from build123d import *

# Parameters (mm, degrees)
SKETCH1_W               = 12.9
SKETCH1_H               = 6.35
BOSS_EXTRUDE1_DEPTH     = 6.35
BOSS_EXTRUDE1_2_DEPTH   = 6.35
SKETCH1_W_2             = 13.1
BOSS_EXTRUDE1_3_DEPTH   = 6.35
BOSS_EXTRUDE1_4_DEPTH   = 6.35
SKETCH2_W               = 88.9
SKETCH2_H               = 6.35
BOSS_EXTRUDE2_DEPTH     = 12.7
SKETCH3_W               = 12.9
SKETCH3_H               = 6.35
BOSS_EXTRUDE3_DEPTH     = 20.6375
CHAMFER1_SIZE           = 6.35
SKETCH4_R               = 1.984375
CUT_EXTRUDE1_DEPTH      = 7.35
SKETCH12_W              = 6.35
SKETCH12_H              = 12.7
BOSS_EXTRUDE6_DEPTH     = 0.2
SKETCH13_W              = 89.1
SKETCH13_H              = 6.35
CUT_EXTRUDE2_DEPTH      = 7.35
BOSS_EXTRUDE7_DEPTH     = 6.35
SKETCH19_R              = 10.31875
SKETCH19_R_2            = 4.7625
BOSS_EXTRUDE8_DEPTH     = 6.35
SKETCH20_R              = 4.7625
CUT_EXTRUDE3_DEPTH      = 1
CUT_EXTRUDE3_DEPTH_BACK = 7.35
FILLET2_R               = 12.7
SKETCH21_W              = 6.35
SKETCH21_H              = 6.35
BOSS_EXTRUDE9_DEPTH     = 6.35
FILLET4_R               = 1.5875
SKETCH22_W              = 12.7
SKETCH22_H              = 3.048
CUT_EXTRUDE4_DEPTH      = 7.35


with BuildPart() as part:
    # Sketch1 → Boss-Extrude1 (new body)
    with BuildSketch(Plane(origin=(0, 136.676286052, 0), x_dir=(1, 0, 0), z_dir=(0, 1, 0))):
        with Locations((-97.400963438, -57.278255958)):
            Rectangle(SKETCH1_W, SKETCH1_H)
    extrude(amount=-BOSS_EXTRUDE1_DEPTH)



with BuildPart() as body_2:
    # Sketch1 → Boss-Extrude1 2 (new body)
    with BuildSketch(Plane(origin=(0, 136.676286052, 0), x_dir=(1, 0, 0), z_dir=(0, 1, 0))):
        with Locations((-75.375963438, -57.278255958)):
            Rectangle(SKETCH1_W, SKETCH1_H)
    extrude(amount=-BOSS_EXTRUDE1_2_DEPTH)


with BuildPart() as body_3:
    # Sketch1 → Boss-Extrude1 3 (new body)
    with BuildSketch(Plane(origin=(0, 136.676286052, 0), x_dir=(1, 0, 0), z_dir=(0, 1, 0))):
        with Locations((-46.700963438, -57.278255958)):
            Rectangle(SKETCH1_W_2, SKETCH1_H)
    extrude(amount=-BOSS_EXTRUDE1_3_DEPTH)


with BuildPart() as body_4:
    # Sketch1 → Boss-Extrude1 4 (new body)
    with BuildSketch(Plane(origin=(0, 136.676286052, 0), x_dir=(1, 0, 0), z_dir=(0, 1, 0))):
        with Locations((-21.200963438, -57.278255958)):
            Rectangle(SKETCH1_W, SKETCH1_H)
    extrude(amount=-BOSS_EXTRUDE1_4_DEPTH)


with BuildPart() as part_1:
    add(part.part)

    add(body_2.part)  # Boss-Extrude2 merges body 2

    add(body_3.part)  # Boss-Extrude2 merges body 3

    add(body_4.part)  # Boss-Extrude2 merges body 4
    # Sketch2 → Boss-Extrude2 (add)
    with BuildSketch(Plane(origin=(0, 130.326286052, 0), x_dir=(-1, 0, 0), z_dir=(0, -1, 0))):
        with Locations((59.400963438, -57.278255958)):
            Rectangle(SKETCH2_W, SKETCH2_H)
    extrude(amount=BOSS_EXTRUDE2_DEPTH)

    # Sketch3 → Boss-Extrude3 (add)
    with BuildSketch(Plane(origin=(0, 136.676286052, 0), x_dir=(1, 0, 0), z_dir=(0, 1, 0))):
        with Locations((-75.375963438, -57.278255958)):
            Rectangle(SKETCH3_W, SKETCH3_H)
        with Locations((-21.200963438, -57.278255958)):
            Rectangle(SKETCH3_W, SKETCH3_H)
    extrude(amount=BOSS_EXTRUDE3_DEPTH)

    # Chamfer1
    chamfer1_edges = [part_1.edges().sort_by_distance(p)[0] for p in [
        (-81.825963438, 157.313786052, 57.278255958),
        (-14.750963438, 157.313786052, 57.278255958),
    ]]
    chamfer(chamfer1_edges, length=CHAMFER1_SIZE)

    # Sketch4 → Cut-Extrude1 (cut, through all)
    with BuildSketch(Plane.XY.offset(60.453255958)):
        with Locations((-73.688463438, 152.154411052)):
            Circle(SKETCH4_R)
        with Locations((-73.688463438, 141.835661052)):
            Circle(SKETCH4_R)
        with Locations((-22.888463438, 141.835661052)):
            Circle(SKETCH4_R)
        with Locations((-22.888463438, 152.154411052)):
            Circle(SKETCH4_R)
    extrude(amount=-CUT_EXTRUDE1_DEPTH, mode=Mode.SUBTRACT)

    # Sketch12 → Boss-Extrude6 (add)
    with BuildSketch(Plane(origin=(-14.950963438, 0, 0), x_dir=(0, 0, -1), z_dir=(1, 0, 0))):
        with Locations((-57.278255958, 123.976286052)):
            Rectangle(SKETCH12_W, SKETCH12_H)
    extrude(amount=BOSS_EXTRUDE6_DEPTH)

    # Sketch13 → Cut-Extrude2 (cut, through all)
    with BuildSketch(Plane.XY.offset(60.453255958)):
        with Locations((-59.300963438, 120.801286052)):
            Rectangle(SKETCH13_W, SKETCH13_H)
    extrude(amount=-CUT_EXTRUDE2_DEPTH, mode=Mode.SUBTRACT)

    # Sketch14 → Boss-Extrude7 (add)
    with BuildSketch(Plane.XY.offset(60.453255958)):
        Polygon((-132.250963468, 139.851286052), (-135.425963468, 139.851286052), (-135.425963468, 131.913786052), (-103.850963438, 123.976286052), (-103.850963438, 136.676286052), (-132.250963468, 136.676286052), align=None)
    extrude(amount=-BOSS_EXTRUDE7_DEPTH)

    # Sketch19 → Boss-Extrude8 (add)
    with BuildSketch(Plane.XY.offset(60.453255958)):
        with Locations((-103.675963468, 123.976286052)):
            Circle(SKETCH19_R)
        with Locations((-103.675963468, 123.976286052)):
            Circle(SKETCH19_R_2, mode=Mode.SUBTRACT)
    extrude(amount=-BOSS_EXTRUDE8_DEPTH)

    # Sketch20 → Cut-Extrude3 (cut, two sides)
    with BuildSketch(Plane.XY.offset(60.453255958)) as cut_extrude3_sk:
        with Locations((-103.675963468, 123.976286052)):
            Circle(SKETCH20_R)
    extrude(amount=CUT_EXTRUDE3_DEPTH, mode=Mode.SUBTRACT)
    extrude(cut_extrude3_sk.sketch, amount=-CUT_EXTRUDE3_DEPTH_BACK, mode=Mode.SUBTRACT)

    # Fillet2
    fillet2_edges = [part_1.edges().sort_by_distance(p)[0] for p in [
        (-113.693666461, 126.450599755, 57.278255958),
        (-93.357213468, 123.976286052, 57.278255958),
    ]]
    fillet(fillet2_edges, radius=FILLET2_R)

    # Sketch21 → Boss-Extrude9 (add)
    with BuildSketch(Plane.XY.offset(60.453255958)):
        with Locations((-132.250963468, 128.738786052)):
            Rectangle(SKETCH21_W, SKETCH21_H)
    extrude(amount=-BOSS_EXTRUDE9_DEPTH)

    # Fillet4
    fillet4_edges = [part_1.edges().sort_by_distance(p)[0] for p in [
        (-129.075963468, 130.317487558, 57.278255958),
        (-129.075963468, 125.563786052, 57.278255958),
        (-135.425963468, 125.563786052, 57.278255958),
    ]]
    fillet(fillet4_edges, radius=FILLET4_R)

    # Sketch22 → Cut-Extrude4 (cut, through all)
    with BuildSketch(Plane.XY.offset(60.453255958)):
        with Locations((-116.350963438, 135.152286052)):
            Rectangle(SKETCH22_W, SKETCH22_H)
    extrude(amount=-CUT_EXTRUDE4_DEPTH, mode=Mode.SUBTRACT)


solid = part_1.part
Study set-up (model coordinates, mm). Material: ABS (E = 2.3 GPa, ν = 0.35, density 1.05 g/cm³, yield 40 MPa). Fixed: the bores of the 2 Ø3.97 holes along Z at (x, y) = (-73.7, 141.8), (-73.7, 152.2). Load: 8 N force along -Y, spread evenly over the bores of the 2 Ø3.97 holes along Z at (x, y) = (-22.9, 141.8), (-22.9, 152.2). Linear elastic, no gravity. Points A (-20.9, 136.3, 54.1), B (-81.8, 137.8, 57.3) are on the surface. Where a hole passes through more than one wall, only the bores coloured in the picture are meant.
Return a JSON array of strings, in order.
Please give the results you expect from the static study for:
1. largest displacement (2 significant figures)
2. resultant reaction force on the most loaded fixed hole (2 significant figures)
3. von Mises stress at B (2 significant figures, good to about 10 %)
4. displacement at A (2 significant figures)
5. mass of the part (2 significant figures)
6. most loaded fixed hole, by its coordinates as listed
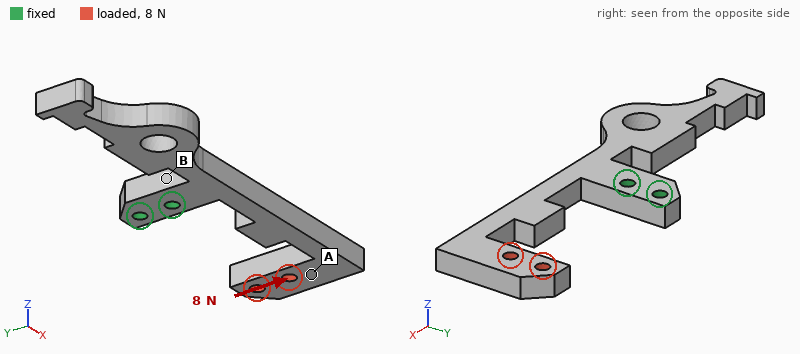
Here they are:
["1.5 mm", "28 N", "2.3 MPa", "1.1 mm", "12 g", "(-73.7, 141.8)"]
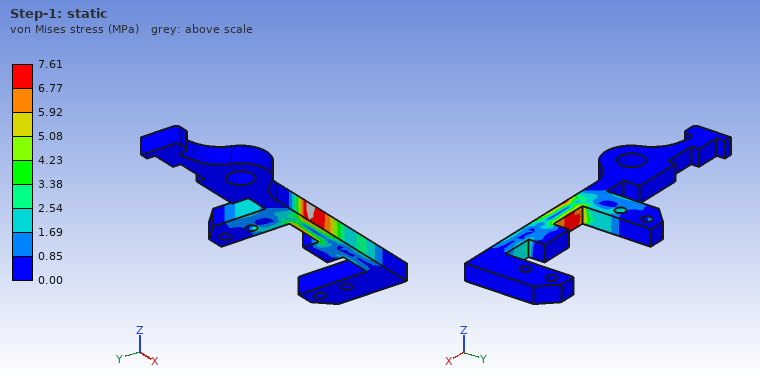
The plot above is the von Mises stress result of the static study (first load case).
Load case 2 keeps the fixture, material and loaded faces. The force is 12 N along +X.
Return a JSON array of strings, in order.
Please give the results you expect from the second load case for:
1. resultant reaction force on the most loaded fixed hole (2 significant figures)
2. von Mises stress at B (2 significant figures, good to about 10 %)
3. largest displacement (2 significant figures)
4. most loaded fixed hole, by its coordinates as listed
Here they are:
["8.8 N", "0.62 MPa", "1.3 mm", "(-73.7, 141.8)"]
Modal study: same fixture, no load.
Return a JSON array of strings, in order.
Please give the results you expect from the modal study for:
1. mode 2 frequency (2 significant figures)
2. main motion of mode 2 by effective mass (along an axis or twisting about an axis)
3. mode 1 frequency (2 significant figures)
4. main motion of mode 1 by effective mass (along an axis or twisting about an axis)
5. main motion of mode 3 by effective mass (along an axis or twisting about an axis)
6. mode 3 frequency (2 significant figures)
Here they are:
["220 Hz", "along Y", "190 Hz", "along Z", "along Z", "320 Hz"]
